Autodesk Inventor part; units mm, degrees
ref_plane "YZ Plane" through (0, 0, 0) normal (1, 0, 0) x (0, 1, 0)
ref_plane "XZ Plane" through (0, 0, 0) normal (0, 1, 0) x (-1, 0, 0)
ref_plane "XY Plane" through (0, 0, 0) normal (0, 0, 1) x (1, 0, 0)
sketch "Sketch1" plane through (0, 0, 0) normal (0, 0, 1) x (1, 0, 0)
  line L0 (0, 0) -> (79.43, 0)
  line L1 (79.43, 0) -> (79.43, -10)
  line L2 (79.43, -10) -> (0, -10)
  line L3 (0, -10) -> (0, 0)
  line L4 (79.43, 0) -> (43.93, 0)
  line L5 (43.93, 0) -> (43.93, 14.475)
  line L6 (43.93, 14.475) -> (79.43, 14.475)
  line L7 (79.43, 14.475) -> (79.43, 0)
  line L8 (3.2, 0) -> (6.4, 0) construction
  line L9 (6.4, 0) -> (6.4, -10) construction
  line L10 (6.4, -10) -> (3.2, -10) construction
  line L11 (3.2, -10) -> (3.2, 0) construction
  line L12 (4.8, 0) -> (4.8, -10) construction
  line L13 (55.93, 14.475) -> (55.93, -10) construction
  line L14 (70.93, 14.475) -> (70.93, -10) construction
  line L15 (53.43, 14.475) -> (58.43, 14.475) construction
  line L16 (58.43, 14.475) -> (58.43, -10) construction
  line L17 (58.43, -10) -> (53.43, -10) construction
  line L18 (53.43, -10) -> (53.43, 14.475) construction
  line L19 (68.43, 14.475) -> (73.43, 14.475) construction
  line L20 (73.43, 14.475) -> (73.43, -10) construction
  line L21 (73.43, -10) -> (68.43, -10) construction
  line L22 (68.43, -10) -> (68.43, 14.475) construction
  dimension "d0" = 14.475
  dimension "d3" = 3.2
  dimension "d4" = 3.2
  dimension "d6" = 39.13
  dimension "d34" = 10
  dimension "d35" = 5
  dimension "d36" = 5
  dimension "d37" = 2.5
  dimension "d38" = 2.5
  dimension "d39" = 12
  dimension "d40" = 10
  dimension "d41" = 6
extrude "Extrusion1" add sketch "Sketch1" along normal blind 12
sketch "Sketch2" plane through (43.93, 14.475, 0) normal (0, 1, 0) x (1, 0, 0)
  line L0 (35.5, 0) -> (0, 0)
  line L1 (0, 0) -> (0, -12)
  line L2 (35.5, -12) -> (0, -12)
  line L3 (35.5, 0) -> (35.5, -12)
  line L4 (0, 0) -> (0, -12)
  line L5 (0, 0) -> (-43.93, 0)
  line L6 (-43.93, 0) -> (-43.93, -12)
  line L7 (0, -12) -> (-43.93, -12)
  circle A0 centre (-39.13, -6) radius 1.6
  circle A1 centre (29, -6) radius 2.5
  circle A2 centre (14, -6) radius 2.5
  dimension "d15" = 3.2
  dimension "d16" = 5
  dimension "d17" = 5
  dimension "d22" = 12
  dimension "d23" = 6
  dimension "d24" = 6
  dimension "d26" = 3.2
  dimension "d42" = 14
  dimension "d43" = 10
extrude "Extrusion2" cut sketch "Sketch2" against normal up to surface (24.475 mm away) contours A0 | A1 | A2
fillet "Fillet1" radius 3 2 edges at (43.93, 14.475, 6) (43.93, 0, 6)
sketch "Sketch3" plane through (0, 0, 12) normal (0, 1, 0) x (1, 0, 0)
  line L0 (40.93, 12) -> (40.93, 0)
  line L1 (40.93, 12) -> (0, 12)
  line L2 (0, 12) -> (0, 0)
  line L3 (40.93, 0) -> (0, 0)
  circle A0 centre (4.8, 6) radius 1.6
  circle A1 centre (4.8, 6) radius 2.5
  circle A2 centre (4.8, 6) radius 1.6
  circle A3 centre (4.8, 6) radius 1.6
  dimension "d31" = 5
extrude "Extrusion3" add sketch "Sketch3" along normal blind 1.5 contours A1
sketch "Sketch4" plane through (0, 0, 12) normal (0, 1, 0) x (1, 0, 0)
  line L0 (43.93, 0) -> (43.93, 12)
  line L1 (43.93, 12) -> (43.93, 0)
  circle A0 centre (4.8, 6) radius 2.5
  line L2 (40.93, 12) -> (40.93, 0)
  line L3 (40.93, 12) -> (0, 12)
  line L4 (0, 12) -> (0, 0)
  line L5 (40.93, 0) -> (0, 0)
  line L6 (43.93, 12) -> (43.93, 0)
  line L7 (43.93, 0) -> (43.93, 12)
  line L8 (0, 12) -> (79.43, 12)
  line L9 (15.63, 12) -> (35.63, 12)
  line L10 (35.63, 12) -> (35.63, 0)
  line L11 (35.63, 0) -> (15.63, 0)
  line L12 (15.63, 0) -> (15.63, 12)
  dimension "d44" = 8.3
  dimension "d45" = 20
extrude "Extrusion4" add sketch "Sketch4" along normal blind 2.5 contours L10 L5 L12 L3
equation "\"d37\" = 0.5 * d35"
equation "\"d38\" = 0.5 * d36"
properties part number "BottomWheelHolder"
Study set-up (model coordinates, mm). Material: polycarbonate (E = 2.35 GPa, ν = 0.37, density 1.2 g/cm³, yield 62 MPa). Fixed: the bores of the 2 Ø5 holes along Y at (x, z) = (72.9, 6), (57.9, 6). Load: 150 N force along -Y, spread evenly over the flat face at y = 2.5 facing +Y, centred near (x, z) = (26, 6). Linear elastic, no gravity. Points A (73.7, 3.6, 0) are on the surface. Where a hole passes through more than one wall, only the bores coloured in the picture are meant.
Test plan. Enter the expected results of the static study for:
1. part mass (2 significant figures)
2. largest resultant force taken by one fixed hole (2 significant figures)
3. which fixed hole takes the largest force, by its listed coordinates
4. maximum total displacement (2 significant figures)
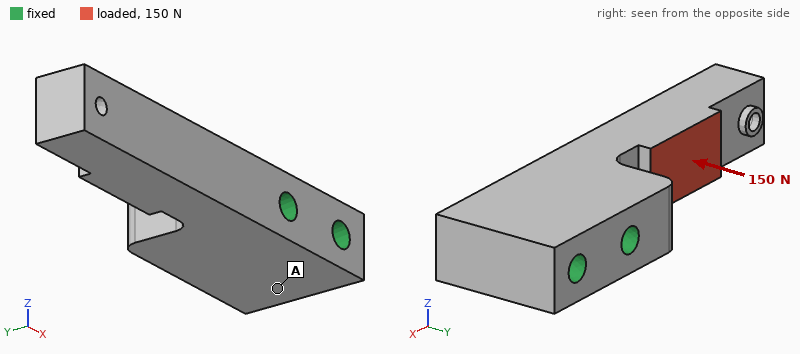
18 g
160 N
(57.9, 6)
0.70 mm
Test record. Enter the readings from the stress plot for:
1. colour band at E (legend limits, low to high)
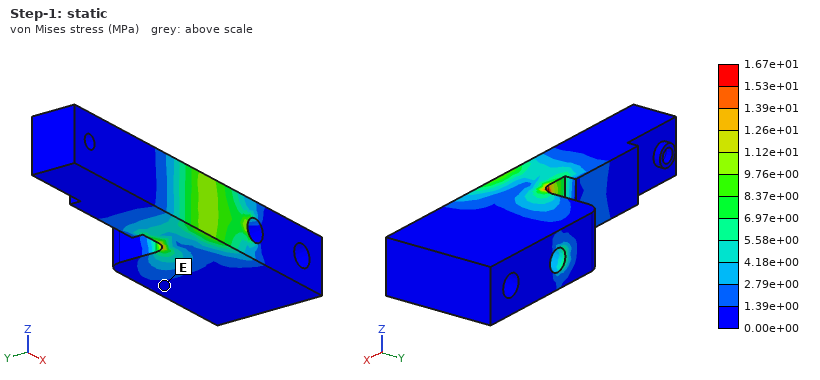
0.00e+00 to 1.39e+00 MPa
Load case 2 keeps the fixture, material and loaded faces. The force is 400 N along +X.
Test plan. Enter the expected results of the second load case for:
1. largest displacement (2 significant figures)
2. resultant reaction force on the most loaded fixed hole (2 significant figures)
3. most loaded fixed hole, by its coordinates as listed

0.83 mm
380 N
(57.9, 6)
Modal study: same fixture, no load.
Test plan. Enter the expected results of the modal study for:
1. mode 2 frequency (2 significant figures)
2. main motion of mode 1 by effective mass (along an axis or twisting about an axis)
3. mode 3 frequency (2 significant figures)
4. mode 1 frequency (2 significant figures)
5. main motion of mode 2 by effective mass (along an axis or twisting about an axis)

970 Hz
along Z
3900 Hz
870 Hz
along Y
